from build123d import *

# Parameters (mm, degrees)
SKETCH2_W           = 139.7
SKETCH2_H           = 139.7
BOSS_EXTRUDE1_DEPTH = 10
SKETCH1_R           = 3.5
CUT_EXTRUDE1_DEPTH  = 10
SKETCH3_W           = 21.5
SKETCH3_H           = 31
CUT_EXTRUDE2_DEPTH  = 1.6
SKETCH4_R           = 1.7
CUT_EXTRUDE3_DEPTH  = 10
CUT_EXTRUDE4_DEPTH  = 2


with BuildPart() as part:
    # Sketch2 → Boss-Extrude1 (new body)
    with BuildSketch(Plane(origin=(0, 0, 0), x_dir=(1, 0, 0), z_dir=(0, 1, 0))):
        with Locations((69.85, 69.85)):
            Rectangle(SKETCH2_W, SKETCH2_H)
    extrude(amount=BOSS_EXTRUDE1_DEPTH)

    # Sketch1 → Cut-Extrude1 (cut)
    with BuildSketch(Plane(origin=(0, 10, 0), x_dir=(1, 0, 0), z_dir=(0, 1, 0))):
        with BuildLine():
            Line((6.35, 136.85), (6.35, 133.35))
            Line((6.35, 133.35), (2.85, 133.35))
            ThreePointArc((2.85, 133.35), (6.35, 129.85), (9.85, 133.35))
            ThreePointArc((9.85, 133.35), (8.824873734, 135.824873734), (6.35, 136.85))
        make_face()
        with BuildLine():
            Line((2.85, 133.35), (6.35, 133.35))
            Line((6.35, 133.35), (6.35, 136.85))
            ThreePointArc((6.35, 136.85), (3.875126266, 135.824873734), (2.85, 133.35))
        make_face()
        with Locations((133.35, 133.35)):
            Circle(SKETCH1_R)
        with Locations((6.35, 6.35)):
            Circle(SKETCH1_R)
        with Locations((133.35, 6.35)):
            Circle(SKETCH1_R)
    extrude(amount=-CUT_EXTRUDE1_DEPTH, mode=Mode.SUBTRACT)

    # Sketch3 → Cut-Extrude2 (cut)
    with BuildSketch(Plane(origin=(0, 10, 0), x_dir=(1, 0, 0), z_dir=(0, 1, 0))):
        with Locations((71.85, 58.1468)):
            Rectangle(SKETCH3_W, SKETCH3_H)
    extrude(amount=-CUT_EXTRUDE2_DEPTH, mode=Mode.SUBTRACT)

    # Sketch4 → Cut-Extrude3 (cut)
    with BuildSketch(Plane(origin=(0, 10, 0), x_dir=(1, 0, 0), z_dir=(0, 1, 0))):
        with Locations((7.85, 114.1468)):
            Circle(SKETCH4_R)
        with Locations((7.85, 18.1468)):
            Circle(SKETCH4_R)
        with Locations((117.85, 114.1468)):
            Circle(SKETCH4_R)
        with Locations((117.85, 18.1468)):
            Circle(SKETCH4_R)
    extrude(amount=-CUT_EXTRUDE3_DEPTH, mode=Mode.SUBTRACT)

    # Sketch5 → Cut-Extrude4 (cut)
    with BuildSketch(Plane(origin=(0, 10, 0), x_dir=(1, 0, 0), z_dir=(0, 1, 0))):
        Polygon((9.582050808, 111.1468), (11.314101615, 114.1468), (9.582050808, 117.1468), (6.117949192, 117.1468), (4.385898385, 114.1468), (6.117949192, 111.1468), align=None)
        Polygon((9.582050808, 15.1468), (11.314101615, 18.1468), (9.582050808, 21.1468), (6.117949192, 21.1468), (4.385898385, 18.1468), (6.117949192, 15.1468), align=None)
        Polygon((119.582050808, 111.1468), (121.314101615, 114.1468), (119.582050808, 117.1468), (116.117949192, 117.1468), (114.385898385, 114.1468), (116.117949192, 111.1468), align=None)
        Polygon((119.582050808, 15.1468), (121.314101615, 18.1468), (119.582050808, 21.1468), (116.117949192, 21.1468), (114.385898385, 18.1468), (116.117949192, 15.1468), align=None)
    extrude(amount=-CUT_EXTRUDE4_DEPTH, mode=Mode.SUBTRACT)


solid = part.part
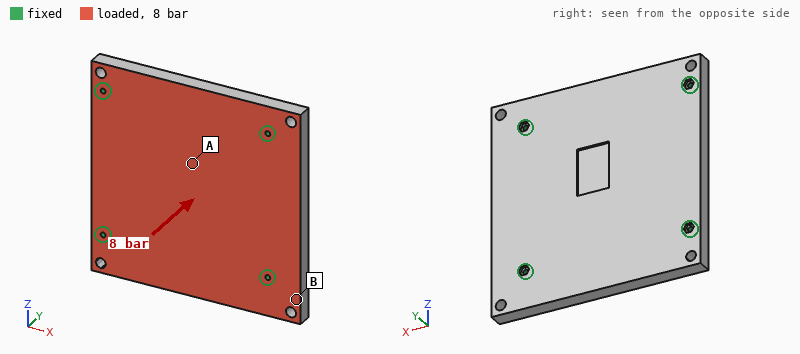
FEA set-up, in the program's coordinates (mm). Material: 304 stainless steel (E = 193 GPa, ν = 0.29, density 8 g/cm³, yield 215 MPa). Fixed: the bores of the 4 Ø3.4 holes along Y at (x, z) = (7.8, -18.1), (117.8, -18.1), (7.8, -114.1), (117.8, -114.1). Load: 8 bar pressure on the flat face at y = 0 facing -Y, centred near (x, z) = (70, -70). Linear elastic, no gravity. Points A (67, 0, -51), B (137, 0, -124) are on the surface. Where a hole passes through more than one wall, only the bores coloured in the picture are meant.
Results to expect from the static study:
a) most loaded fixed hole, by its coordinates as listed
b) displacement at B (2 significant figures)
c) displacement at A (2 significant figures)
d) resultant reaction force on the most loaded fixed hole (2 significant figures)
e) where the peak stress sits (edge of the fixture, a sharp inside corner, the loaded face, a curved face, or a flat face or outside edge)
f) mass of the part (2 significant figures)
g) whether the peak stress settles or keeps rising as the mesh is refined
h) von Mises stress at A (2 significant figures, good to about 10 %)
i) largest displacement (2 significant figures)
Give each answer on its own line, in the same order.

(117.8, -114.1)
13 µm
61 µm
4.7 kN
edge of the fixture
1.5 kg
keeps rising
37 MPa
63 µm
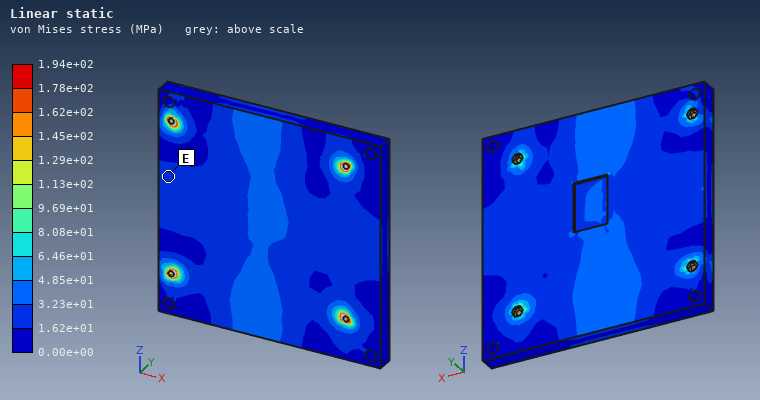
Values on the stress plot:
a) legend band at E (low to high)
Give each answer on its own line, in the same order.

1.62e+01 to 3.23e+01 MPa
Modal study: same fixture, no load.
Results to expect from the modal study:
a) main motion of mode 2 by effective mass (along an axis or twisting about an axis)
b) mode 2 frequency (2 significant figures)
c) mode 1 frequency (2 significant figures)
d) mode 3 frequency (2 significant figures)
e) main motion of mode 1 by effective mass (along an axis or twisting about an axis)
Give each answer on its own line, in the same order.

twisting about X
3200 Hz
2400 Hz
3600 Hz
along Y
